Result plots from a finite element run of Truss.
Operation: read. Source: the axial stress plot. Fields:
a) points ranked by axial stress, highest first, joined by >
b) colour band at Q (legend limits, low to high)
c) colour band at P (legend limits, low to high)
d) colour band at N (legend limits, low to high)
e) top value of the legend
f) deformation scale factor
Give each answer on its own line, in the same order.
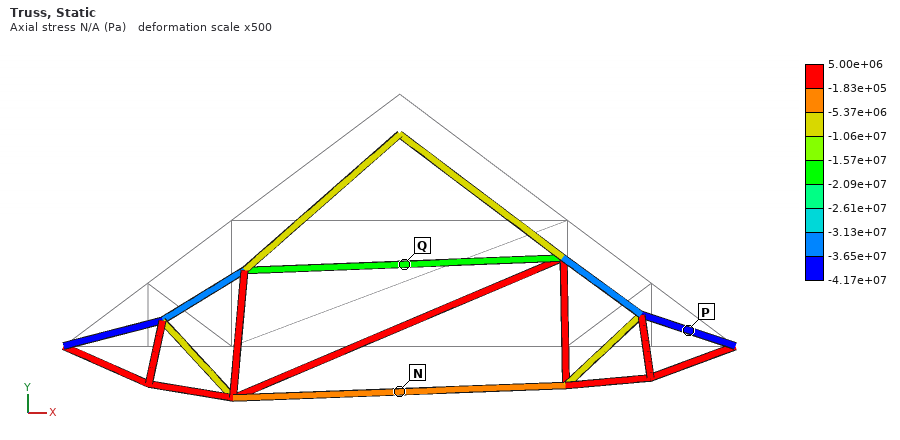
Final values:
N > Q > P
-2.09e+07 to -1.57e+07 Pa
-4.17e+07 to -3.65e+07 Pa
-5.37e+06 to -1.83e+05 Pa
5.00e+06 Pa
500
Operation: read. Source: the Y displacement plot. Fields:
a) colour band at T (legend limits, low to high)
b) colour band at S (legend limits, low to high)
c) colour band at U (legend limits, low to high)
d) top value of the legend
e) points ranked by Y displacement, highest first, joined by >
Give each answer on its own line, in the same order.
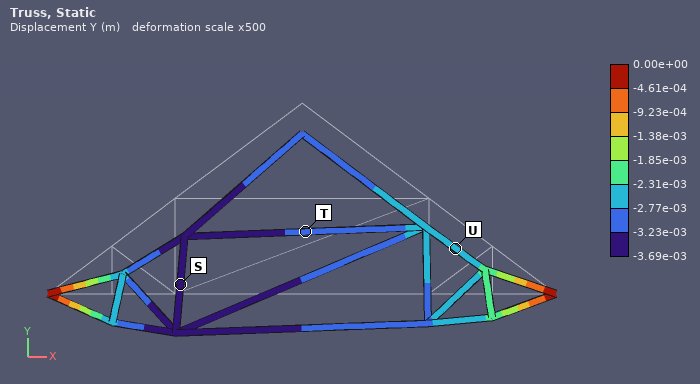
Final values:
-3.23e-03 to -2.77e-03 m
-3.69e-03 to -3.23e-03 m
-2.77e-03 to -2.31e-03 m
0.00e+00 m
U > T > S
